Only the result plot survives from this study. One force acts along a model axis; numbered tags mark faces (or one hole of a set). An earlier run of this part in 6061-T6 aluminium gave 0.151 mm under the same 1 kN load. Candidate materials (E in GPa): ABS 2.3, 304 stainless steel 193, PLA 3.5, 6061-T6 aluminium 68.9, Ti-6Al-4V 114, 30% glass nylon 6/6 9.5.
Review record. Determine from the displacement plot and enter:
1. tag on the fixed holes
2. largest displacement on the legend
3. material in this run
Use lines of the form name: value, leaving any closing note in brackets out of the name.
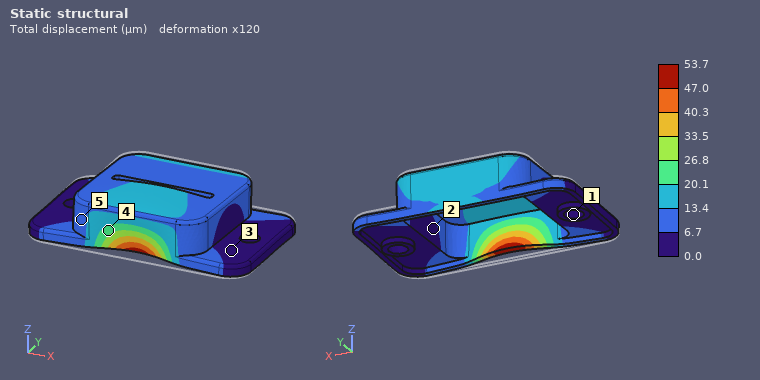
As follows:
tag on the fixed holes: 1
largest displacement on the legend: 53.7 µm
material in this run: 304 stainless steel
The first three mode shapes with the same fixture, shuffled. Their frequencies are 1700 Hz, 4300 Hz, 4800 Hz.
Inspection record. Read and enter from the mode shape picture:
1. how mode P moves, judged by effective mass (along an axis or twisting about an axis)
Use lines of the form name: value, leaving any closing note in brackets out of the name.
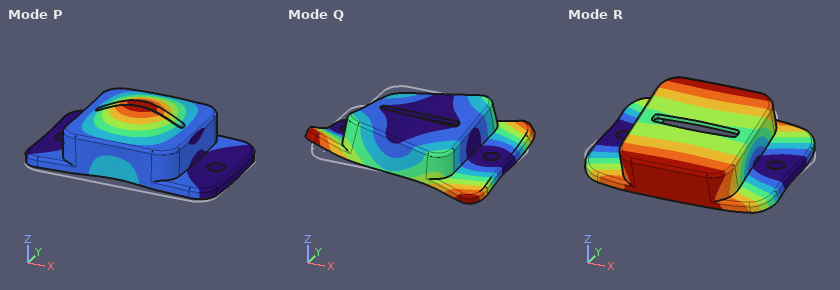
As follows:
how mode P moves, judged by effective mass: along Z
